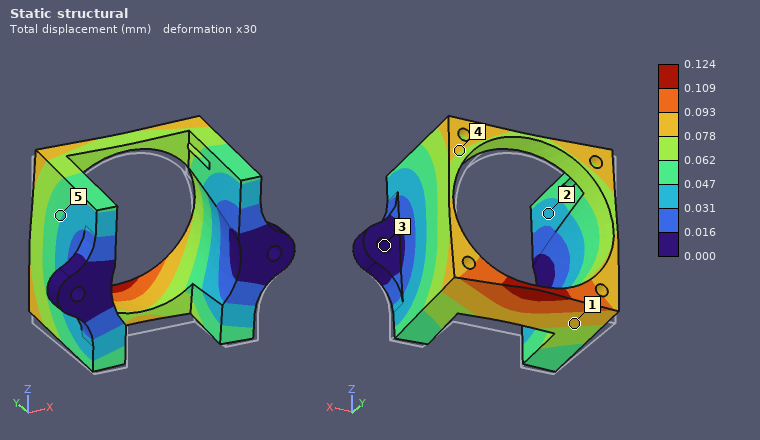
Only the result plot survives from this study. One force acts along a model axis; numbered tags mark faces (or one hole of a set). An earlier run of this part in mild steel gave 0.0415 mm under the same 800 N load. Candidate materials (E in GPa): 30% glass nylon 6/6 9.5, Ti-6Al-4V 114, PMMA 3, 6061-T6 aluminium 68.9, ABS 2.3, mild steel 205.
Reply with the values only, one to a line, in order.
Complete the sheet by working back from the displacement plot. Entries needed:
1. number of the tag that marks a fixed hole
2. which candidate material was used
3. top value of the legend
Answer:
3
6061-T6 aluminium
0.124 mm
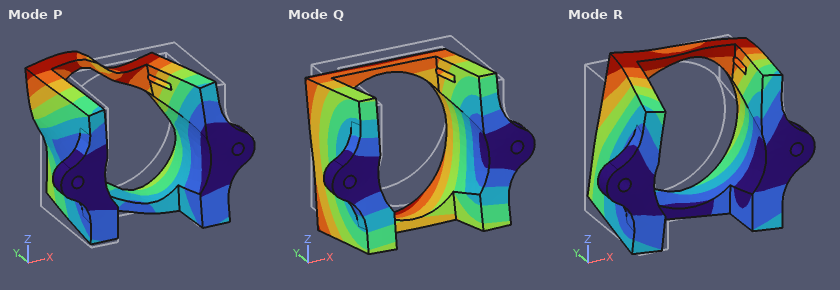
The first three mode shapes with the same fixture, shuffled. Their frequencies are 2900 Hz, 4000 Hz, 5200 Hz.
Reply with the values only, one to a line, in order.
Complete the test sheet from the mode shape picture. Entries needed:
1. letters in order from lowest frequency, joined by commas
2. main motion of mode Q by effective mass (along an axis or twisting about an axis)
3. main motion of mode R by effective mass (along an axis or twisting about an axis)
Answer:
Q, R, P
along Z
along X
